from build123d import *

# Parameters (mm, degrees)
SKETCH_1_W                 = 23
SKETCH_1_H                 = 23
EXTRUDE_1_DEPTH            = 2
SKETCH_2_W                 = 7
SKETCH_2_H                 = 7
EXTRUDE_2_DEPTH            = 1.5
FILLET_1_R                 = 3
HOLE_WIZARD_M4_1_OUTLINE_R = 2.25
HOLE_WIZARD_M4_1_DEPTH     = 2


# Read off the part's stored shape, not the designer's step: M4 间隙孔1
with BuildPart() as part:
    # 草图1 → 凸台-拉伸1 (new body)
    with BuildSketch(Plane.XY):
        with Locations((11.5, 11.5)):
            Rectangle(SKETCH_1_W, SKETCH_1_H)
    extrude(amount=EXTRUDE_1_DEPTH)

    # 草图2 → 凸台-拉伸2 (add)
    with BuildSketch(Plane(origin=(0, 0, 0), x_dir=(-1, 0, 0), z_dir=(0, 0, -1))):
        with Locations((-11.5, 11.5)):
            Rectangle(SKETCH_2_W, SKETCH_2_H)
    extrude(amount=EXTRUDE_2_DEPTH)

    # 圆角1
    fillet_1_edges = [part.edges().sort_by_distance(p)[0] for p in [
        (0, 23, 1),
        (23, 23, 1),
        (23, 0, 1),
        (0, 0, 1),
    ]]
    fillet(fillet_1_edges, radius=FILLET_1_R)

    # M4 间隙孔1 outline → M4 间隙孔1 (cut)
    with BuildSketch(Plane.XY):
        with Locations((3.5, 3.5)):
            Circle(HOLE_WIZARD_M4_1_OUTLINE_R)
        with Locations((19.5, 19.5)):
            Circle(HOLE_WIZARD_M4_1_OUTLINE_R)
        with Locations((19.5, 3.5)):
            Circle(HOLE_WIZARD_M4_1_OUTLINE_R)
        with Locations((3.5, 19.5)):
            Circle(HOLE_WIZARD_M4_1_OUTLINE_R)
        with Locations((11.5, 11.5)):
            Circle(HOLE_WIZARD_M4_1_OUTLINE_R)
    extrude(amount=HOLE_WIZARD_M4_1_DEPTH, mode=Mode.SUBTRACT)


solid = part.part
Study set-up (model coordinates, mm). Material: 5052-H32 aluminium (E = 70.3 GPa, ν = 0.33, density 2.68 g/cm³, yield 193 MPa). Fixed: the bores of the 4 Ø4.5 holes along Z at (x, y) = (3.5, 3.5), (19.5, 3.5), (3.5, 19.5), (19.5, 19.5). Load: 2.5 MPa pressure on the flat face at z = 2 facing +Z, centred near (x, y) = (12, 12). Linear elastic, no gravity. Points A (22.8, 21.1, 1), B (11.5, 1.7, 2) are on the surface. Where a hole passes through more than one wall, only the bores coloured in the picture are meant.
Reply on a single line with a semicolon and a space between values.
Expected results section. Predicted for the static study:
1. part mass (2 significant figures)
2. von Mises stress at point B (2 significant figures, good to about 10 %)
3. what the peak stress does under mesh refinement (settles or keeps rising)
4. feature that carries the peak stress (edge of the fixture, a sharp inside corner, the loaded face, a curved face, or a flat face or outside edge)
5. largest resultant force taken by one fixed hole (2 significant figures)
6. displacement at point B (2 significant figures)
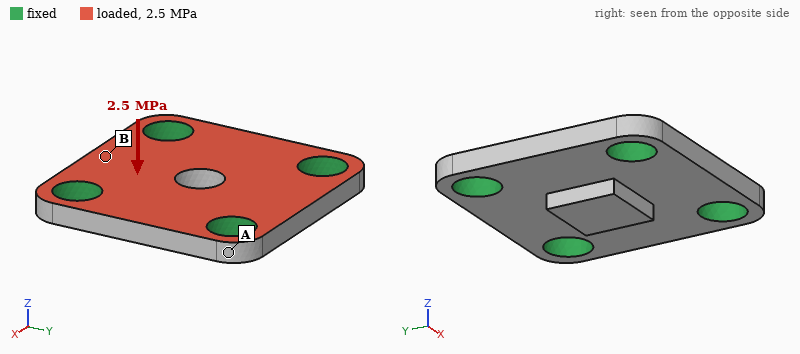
2.6 g; 24 MPa; keeps rising; edge of the fixture; 280 N; 4.4 µm
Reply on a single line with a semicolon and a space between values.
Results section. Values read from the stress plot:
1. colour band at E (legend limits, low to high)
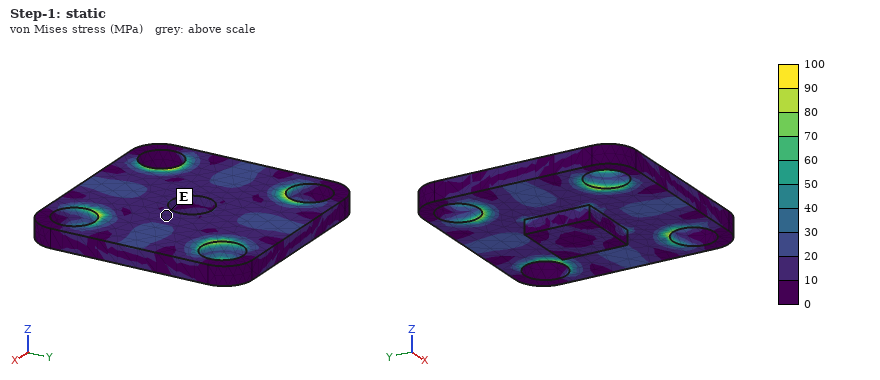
10 to 20 MPa
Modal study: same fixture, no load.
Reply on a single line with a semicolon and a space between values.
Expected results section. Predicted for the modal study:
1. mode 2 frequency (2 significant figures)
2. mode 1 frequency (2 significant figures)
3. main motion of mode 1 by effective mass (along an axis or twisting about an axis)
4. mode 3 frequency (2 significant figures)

60 kHz; 42 kHz; along Z; 60 kHz
